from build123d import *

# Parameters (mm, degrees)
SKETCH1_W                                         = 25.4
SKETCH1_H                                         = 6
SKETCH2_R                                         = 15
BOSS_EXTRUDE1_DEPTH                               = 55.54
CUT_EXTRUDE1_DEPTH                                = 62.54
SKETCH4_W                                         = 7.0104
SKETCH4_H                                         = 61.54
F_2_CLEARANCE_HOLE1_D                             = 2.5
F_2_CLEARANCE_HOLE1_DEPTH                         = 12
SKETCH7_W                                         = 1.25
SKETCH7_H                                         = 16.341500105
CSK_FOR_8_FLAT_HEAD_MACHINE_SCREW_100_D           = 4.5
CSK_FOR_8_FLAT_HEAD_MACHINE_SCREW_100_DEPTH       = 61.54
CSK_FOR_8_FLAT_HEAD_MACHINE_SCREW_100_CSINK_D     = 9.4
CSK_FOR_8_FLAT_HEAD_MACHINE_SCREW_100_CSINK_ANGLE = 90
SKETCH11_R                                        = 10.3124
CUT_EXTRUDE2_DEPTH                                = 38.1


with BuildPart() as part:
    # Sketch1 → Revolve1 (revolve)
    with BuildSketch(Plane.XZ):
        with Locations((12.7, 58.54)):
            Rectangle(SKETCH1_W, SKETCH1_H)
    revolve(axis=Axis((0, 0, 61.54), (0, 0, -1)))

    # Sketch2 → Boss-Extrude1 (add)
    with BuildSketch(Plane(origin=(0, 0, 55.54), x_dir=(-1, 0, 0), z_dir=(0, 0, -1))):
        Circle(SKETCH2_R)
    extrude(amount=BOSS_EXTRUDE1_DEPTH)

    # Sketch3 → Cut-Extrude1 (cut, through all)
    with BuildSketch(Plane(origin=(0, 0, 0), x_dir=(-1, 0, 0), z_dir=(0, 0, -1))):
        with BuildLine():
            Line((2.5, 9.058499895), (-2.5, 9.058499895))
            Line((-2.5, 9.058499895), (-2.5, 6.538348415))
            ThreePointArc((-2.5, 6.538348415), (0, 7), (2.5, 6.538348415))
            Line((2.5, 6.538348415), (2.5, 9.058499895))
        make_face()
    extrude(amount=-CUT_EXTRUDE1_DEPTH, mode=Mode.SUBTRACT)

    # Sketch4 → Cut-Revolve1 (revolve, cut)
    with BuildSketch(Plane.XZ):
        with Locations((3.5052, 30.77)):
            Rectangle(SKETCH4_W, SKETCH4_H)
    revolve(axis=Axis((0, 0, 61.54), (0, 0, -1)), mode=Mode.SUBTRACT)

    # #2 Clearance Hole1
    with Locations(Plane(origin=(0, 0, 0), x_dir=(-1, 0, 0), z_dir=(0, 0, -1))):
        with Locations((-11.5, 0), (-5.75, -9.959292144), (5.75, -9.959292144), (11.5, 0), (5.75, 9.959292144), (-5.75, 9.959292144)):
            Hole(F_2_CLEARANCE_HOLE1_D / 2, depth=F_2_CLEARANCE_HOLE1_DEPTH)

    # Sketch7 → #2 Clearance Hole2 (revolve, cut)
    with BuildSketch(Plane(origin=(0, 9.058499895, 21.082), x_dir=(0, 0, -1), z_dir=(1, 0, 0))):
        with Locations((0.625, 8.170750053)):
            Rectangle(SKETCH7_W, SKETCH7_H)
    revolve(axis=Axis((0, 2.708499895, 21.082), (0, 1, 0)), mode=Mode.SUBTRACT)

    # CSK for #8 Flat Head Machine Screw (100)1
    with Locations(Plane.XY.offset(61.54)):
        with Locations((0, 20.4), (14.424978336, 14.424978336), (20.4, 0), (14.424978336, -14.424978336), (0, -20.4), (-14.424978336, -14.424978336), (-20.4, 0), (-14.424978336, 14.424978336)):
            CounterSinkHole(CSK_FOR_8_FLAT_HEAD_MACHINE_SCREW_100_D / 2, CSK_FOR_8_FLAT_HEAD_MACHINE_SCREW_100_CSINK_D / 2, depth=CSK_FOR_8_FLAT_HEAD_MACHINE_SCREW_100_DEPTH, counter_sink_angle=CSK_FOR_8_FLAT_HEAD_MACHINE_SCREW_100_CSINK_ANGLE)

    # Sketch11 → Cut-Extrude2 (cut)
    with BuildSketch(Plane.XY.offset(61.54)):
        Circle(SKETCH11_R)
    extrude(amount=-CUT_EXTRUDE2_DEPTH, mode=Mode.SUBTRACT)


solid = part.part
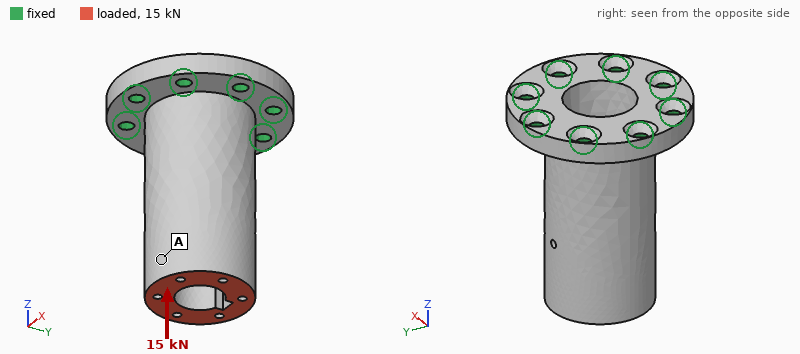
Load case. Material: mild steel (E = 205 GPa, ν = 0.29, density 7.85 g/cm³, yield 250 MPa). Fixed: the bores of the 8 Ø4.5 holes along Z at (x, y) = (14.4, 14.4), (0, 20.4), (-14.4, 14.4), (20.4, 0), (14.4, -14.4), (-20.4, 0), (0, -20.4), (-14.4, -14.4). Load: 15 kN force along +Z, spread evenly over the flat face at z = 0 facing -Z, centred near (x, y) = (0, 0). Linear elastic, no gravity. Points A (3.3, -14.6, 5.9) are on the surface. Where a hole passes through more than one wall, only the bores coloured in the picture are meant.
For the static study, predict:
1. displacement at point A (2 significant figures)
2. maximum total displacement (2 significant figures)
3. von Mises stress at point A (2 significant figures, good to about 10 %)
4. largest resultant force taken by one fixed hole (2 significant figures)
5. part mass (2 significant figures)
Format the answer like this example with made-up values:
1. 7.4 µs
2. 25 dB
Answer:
1. 15 µm
2. 16 µm
3. 29 MPa
4. 1.9 kN
5. 260 g
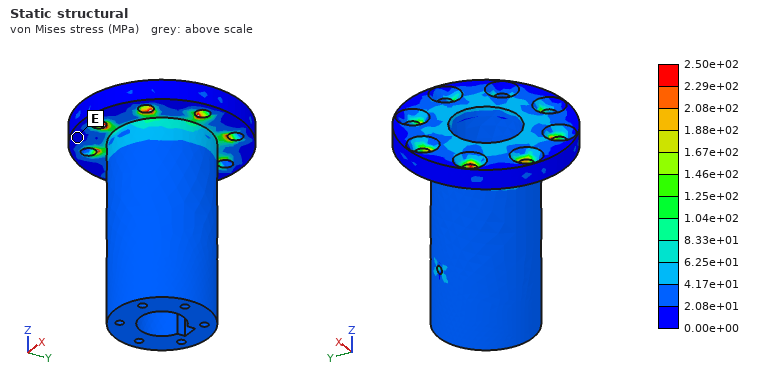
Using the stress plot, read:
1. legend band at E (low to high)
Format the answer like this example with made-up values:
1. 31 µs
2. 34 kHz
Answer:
1. 0.00e+00 to 2.08e+01 MPa
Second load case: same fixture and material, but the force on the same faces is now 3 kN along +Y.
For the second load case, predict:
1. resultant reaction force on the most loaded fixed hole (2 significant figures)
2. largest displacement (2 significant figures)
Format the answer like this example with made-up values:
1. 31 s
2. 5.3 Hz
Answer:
1. 2.5 kN
2. 63 µm
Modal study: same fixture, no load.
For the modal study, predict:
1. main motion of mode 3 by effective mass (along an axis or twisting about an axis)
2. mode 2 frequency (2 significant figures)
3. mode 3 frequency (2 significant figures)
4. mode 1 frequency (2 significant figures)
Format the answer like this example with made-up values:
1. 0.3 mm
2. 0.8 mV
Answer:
1. twisting about Z
2. 4300 Hz
3. 13 kHz
4. 4300 Hz
